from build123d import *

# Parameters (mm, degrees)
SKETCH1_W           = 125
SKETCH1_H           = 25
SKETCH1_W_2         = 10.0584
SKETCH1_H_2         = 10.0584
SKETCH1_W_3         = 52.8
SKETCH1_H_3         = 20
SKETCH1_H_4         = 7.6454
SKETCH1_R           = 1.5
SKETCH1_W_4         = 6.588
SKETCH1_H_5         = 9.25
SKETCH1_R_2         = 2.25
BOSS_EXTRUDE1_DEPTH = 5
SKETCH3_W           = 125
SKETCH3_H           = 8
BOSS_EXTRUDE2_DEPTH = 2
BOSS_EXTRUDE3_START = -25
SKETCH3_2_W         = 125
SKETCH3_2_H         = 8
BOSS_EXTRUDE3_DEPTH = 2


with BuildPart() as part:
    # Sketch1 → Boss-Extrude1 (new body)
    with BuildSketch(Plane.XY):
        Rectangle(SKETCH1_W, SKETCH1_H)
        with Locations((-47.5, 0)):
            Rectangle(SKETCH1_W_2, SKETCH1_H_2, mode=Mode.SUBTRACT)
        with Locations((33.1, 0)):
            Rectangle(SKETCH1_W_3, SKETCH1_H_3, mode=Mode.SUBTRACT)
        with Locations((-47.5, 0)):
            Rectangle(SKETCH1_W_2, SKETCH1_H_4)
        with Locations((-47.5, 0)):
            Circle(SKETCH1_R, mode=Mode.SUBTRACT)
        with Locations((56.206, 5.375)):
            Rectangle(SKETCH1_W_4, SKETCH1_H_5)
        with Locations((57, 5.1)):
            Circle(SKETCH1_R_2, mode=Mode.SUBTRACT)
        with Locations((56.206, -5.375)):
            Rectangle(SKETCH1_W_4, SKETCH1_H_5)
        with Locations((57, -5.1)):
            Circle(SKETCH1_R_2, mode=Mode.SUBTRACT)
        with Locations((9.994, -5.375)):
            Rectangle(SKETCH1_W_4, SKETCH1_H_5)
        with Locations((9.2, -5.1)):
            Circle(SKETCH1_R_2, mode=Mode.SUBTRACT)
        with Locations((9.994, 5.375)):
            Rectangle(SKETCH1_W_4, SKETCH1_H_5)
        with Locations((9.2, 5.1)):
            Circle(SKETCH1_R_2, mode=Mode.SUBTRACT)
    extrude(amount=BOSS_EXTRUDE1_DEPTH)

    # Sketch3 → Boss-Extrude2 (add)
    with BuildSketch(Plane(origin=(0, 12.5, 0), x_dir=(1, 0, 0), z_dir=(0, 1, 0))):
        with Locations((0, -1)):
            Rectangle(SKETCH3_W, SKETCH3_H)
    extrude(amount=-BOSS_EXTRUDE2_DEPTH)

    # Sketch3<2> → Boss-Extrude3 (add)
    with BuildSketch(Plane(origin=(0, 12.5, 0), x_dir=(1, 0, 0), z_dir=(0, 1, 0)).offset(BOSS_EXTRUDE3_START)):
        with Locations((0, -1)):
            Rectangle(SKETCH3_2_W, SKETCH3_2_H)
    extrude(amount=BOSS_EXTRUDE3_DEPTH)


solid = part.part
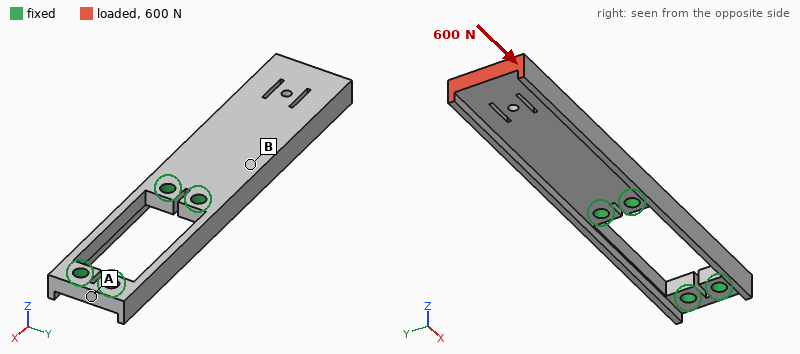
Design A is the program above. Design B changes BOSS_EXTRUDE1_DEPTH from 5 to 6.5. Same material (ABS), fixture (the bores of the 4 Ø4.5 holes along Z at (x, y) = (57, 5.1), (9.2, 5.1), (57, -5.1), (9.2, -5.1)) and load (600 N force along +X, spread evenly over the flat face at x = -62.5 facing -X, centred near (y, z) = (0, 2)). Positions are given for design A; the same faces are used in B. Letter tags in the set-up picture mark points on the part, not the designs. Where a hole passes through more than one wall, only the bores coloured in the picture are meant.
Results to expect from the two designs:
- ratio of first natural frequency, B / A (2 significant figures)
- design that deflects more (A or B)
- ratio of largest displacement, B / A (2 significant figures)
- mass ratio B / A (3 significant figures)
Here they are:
1.2
A
0.71
1.26
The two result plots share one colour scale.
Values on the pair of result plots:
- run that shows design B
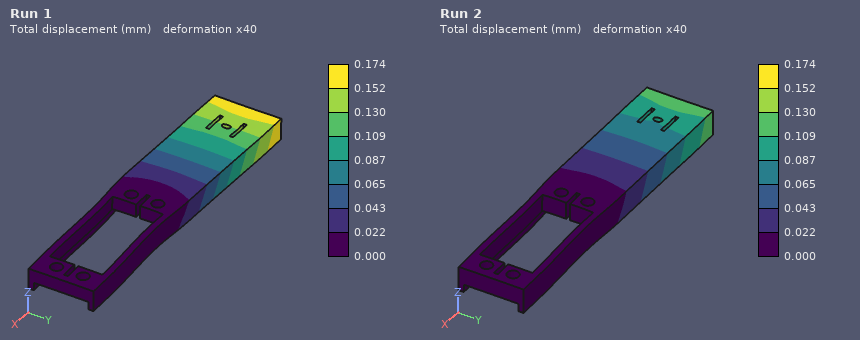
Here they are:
Run 2
